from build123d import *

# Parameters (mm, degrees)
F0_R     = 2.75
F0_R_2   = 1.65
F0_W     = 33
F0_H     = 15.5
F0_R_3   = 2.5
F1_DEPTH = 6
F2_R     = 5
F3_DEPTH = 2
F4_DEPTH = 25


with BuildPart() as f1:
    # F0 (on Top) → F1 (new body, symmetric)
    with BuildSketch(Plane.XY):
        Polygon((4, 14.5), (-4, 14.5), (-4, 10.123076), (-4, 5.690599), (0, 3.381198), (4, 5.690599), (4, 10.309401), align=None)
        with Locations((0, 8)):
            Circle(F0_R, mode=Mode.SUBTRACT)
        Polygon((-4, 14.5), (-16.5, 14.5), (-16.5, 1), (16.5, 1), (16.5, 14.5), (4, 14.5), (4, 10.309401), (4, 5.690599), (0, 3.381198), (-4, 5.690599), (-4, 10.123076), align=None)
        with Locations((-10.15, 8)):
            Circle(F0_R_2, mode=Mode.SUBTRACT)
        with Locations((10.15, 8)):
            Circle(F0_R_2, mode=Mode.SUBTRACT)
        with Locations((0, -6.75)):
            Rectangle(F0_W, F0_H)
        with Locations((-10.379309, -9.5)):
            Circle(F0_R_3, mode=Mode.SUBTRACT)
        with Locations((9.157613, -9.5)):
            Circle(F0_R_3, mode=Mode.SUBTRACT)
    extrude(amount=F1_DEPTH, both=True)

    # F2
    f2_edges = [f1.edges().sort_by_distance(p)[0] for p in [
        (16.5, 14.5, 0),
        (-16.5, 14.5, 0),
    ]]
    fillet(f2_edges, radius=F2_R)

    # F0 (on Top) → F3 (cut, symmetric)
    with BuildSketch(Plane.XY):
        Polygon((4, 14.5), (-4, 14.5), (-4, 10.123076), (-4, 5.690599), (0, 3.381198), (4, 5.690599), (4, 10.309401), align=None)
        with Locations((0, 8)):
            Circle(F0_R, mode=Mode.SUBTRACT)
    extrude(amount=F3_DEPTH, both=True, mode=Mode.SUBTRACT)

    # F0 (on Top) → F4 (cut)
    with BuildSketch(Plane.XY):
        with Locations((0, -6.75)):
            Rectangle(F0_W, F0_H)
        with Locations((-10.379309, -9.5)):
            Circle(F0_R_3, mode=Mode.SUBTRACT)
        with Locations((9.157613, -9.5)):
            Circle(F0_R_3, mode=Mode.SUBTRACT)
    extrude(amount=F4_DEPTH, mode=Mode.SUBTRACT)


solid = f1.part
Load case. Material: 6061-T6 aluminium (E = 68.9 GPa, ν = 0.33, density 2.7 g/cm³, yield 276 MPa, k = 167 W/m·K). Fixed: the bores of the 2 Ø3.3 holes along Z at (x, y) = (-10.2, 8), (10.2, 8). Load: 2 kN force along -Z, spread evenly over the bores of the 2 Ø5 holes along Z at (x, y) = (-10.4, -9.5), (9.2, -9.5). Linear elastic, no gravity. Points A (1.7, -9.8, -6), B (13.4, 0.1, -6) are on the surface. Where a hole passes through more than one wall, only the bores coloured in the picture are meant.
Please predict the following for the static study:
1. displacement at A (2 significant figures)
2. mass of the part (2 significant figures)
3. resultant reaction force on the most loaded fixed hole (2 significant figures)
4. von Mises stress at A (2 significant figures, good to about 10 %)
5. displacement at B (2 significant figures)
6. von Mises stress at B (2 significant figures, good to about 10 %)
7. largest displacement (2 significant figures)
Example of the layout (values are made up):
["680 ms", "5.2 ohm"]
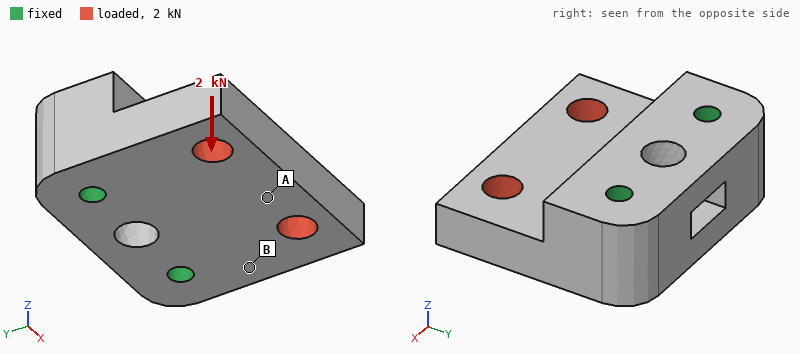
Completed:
["56 µm", "20 g", "1.0 kN", "14 MPa", "13 µm", "87 MPa", "83 µm"]
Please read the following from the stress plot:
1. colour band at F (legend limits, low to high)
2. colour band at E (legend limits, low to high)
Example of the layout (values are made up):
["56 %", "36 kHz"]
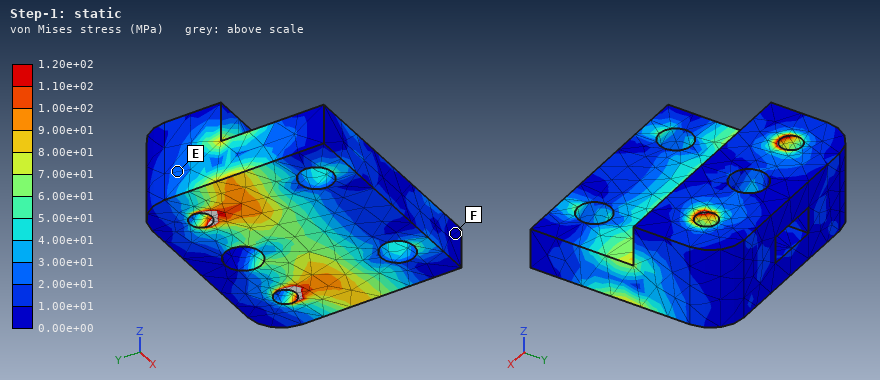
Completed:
["0.00e+00 to 1.00e+01 MPa", "2.00e+01 to 3.00e+01 MPa"]
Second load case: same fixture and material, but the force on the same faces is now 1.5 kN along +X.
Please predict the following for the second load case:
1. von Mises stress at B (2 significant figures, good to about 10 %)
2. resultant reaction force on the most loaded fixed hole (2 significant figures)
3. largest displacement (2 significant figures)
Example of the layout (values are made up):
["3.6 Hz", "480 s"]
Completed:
["9.1 MPa", "1.3 kN", "11 µm"]
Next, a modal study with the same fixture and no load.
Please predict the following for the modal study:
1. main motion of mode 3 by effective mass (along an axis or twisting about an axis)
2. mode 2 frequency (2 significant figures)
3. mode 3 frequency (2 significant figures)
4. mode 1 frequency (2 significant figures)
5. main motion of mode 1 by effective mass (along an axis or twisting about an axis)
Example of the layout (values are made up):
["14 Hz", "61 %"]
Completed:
["along X", "20 kHz", "27 kHz", "13 kHz", "along Z"]
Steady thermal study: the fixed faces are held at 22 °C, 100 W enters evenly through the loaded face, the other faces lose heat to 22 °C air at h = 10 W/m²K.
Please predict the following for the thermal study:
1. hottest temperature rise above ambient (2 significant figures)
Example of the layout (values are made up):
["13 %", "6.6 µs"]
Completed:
["63 K"]
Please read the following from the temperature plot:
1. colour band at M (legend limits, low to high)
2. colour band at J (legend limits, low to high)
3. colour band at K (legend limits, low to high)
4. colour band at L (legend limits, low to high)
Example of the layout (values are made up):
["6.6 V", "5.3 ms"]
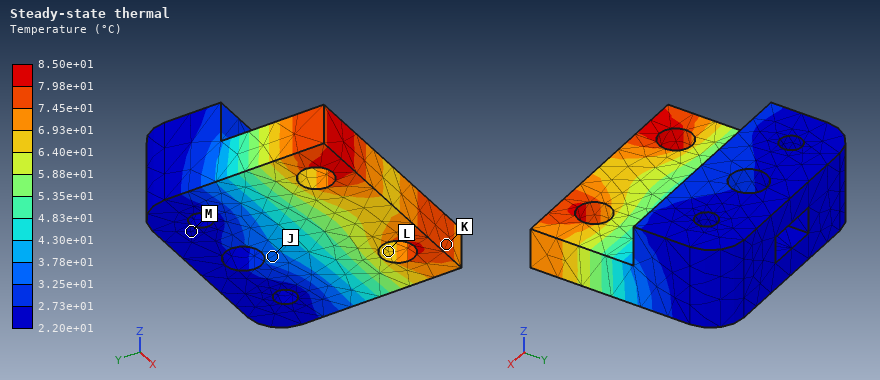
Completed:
["2.20e+01 to 2.73e+01 °C", "3.25e+01 to 3.78e+01 °C", "7.45e+01 to 7.98e+01 °C", "6.40e+01 to 6.93e+01 °C"]
